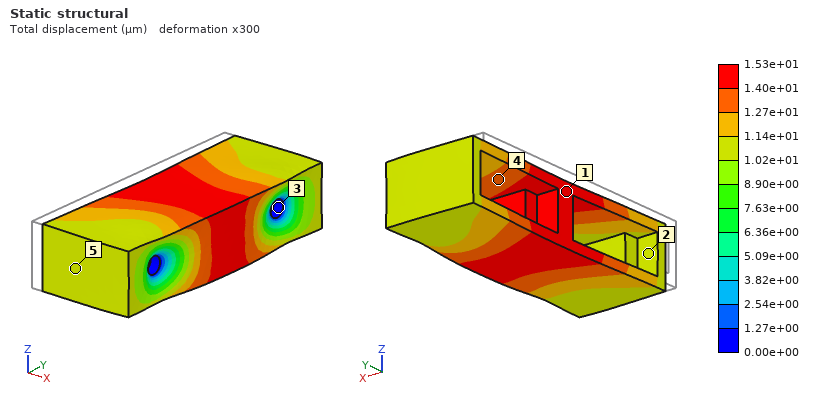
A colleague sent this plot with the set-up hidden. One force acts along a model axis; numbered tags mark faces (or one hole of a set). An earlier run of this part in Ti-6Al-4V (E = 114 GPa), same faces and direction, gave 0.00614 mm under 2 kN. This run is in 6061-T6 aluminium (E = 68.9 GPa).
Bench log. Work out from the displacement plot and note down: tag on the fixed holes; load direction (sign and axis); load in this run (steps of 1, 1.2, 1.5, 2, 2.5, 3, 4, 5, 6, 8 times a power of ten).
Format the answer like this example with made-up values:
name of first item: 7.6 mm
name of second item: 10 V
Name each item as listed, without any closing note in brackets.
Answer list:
tag on the fixed holes: 3
load direction: +X
load in this run: 3 kN
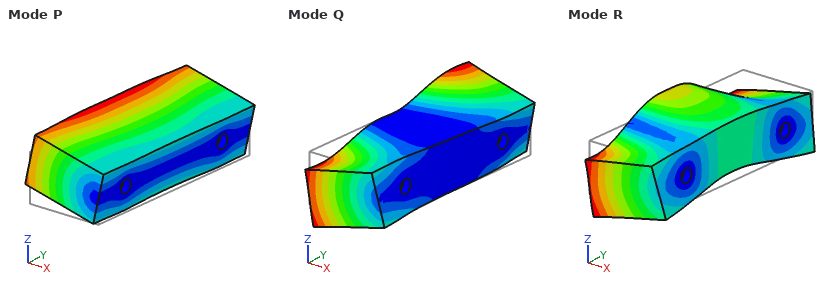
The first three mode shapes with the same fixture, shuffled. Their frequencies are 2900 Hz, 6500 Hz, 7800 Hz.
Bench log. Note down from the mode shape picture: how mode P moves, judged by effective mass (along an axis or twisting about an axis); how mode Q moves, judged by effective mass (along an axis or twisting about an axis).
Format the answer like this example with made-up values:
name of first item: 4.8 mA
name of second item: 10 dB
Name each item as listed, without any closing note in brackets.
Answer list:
how mode P moves, judged by effective mass: along Z
how mode Q moves, judged by effective mass: twisting about X
